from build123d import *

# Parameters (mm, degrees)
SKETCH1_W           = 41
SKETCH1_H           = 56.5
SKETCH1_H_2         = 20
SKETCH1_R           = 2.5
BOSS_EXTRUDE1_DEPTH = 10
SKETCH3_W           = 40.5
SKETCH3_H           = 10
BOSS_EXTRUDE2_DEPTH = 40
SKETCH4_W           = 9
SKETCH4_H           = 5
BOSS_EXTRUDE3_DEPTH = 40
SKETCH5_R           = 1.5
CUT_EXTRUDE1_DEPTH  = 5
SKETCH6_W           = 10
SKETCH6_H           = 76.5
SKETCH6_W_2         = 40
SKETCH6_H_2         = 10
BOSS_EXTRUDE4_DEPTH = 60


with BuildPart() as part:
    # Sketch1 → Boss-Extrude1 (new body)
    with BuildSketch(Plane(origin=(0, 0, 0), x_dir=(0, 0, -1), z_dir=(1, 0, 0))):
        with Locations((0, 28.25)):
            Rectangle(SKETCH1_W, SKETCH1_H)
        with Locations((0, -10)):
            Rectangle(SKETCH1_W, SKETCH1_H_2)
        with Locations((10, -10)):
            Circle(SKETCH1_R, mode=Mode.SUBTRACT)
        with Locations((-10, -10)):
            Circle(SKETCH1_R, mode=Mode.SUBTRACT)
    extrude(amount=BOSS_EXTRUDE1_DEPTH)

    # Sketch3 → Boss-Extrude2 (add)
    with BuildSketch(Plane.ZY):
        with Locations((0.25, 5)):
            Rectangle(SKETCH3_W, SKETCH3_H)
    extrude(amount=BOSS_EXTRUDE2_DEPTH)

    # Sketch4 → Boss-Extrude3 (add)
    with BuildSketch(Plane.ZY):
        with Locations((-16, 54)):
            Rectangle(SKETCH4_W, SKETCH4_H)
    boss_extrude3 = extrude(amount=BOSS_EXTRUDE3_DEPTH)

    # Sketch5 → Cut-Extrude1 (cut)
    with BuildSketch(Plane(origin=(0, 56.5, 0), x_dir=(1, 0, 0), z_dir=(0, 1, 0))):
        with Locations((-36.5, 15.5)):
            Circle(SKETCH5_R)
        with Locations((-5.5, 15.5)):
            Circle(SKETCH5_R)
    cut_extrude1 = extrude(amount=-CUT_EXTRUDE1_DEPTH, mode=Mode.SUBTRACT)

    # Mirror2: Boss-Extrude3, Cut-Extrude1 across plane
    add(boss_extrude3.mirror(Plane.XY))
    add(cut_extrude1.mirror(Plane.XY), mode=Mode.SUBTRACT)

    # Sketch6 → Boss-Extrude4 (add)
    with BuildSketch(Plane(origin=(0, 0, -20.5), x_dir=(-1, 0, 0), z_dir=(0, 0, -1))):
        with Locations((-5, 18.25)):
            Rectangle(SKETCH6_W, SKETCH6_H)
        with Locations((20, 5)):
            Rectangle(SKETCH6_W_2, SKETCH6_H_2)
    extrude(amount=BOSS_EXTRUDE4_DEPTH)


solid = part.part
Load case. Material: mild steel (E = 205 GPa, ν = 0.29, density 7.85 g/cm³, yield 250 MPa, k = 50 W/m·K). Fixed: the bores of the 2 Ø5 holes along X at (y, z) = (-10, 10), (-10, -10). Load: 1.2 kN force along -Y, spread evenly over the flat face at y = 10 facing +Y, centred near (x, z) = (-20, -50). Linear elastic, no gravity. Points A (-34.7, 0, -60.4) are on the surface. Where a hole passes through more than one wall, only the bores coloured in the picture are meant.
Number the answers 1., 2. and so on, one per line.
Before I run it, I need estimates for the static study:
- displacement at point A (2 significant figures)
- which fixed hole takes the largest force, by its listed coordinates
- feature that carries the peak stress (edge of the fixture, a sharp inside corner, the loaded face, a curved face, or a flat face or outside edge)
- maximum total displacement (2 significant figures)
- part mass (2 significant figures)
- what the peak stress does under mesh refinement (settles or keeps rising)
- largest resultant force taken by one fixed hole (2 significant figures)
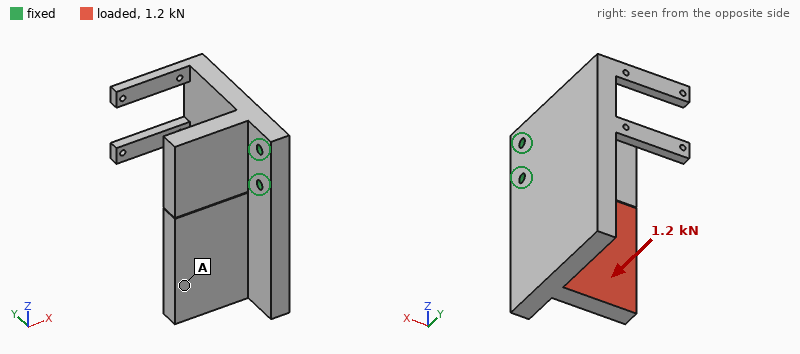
1. 54 µm
2. (-10, -10)
3. edge of the fixture
4. 68 µm
5. 950 g
6. keeps rising
7. 3.1 kN
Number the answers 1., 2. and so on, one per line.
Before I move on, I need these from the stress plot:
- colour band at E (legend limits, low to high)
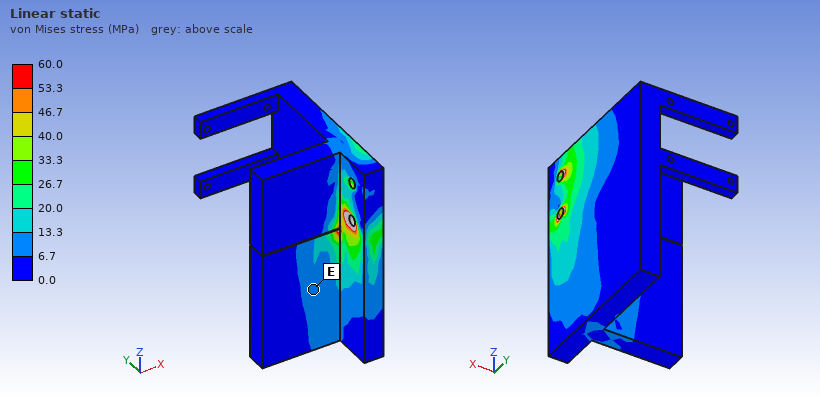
1. 6.7 to 13.3 MPa
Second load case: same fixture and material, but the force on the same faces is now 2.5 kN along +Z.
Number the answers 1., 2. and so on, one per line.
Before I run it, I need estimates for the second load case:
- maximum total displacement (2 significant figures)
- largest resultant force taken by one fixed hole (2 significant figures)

1. 0.12 mm
2. 3.0 kN
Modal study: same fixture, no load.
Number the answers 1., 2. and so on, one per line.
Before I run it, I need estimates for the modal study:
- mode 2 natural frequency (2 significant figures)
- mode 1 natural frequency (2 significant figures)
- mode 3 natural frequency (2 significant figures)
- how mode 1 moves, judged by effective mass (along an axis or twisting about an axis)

1. 1300 Hz
2. 880 Hz
3. 2000 Hz
4. along X
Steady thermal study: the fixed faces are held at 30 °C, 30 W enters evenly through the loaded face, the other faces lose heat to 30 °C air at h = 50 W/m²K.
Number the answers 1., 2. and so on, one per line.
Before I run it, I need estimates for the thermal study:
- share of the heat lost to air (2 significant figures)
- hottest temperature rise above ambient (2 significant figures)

1. 60 %
2. 38 K
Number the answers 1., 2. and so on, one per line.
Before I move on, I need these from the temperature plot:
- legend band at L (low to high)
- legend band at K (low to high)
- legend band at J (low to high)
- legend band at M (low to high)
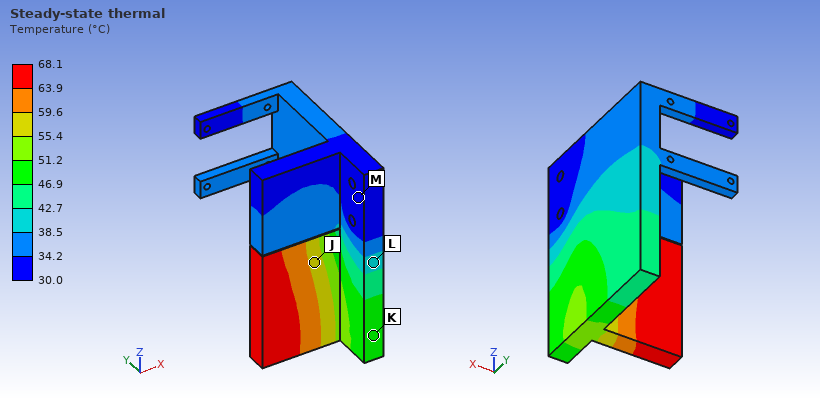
1. 38.5 to 42.7 °C
2. 46.9 to 51.2 °C
3. 55.4 to 59.6 °C
4. 30.0 to 34.2 °C
